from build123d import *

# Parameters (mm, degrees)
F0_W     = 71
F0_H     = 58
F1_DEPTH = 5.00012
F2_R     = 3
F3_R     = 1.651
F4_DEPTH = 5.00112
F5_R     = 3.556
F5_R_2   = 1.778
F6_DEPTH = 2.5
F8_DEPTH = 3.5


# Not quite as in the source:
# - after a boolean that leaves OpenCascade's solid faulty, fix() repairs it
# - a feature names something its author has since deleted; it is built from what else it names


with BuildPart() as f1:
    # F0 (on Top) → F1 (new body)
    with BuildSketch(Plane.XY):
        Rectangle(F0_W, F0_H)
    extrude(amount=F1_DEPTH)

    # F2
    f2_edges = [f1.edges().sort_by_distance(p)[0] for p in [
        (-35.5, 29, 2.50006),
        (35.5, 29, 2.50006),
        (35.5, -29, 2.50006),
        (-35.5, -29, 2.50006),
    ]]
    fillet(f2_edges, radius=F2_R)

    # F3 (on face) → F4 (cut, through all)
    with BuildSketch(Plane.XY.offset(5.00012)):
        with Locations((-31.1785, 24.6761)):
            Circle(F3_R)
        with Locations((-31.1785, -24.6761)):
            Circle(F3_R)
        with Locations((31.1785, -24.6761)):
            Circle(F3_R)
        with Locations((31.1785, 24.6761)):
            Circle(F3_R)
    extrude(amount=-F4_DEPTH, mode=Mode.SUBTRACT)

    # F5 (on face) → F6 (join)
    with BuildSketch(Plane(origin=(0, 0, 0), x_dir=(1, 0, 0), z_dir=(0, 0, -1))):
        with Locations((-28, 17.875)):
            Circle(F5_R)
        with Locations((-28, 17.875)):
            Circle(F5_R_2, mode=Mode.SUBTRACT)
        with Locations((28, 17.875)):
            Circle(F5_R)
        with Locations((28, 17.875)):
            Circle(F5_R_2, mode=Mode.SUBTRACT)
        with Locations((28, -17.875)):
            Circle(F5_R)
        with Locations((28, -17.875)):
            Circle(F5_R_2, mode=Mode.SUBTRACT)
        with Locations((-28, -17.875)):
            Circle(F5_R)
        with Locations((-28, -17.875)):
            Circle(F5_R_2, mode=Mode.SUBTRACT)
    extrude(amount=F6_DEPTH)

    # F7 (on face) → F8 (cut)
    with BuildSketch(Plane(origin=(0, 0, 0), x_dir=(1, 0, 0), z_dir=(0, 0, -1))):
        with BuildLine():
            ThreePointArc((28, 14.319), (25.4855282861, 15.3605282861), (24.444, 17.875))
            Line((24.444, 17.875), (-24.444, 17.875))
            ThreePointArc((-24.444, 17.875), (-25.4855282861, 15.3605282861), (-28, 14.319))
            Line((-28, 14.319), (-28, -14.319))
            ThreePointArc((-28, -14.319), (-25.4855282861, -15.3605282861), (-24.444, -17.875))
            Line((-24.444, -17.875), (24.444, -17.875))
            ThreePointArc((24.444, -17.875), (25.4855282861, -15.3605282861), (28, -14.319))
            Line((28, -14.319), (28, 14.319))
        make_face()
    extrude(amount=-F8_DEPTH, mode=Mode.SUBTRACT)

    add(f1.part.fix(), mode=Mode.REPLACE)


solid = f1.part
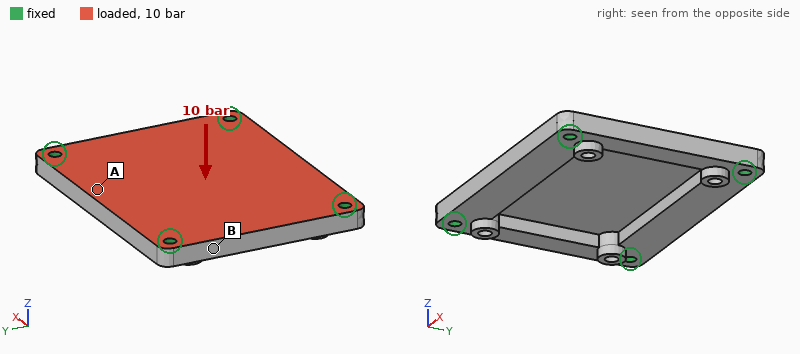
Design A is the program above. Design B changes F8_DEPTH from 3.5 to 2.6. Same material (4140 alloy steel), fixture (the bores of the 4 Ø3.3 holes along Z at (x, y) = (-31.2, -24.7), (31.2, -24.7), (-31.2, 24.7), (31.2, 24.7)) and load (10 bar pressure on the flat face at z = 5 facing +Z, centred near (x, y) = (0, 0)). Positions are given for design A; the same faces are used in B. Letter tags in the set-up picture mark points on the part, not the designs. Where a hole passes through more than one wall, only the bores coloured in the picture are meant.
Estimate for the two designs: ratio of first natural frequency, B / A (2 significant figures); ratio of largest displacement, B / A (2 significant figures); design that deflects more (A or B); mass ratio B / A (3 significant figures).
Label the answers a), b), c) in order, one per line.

a) 0.99
b) 0.60
c) A
d) 1.13
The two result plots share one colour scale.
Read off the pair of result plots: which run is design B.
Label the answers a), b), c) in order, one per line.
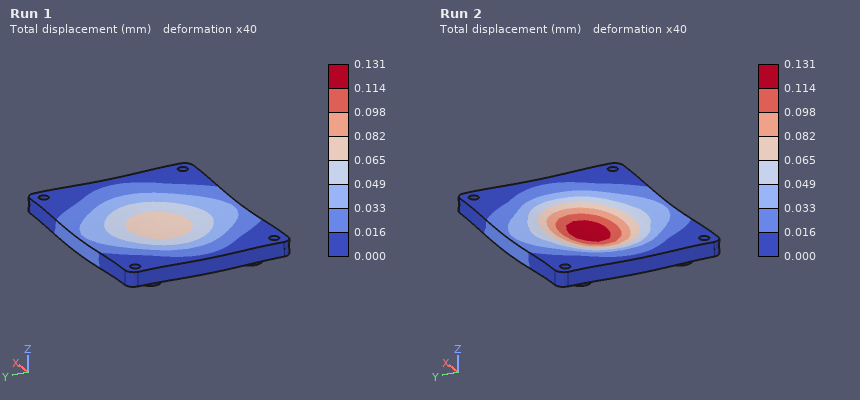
a) Run 1
